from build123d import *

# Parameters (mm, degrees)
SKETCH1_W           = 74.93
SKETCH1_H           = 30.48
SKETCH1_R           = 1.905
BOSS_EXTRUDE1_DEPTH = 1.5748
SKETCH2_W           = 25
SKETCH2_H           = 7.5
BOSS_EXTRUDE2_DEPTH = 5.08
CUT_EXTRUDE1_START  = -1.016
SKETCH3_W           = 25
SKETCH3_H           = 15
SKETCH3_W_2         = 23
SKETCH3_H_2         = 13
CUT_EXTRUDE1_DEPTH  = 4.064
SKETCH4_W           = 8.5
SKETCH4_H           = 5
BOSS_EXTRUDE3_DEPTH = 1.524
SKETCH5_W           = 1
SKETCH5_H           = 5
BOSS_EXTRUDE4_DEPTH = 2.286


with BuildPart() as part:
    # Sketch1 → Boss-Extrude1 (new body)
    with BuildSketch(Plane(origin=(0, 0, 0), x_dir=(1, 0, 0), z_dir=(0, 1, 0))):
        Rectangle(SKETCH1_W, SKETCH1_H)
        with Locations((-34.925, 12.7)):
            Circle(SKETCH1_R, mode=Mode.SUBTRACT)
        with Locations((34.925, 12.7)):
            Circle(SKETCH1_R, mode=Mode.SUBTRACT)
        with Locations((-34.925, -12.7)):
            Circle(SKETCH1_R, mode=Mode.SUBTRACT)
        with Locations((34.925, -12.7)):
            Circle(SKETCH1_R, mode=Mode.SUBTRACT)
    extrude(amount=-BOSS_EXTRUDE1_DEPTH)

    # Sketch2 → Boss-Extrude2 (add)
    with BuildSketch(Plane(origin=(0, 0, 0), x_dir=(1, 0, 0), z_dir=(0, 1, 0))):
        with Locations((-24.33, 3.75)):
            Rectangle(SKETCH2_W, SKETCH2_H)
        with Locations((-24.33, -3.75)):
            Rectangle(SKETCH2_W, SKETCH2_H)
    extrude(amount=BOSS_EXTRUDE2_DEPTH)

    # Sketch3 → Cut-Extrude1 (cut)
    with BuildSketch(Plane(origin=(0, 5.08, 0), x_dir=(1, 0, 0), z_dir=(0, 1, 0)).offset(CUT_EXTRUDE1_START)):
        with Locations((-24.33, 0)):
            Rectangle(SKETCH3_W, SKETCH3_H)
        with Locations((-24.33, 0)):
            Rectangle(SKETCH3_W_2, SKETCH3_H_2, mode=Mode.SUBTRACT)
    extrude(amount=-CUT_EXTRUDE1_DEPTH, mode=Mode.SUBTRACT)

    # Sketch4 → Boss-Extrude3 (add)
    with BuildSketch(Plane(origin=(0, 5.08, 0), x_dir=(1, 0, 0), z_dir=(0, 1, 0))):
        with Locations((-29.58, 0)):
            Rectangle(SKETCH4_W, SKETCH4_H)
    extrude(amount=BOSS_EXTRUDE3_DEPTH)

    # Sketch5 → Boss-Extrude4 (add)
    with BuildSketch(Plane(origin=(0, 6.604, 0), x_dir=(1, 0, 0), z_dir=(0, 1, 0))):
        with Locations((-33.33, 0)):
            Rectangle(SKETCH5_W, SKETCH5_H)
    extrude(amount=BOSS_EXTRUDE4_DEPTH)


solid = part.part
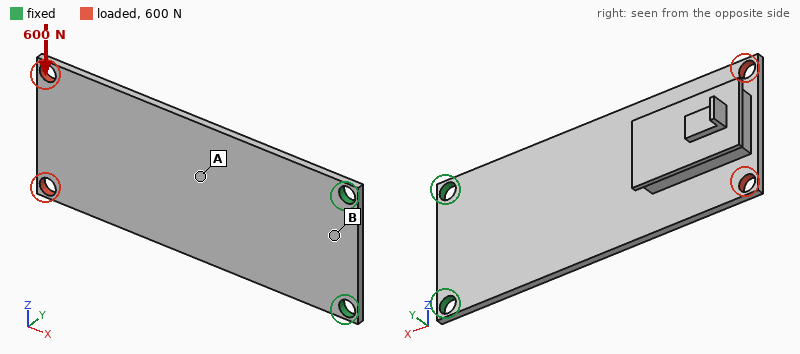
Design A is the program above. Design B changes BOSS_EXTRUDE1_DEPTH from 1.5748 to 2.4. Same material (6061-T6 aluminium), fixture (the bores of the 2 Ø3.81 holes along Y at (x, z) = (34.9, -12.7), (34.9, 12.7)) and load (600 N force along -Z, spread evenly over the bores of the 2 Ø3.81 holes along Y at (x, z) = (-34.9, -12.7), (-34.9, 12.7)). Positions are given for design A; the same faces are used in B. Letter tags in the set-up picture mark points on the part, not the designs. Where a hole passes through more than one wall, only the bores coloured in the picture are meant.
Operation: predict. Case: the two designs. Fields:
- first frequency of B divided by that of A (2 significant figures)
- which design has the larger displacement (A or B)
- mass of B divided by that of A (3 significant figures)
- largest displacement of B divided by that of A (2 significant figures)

1.7
A
1.36
0.66
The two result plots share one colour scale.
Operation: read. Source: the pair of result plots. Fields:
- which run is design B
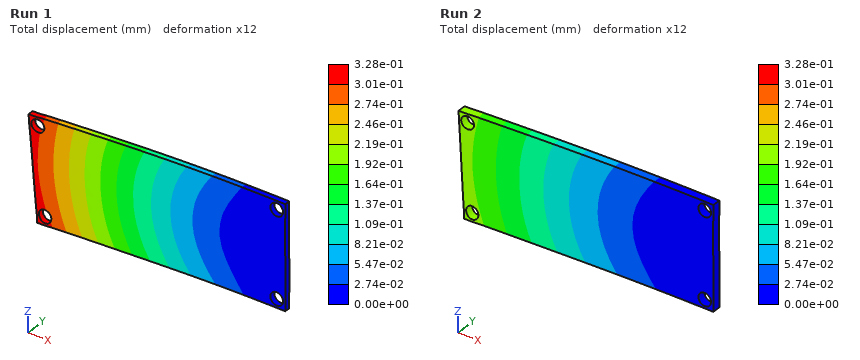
Run 2
